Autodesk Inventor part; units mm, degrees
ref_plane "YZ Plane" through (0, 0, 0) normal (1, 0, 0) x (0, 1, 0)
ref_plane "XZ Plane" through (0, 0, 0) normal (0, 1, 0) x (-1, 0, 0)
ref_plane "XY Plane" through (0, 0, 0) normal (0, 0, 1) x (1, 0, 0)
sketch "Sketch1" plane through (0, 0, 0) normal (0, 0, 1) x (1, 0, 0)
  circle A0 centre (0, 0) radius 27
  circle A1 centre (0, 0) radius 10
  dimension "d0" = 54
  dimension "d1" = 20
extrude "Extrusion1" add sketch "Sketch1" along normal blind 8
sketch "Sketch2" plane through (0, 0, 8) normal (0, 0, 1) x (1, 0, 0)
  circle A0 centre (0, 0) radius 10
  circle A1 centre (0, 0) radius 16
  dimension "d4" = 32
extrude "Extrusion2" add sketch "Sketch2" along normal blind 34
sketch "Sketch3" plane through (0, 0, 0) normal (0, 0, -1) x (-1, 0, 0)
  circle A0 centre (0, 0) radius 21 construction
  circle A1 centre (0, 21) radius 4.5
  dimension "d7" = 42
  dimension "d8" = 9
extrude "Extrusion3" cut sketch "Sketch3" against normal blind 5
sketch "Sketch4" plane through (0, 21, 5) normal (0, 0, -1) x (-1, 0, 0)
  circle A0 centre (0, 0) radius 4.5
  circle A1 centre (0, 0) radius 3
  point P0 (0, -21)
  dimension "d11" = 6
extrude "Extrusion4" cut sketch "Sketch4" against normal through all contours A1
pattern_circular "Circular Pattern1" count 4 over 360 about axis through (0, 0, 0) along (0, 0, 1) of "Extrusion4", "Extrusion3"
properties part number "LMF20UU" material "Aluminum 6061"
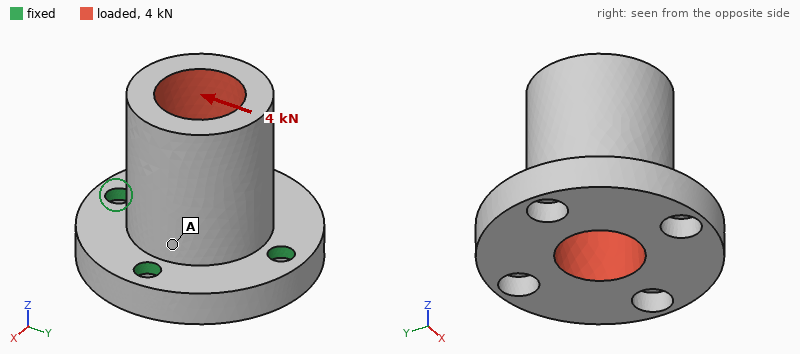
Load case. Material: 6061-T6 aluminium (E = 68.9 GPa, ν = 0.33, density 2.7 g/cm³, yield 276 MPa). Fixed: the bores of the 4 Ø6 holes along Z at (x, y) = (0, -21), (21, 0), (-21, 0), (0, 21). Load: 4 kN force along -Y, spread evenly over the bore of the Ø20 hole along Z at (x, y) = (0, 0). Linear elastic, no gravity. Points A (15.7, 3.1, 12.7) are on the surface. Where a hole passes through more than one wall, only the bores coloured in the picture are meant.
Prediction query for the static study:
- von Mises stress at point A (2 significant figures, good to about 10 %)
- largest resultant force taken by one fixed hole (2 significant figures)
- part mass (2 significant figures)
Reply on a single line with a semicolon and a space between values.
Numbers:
10 MPa; 1.7 kN; 83 g
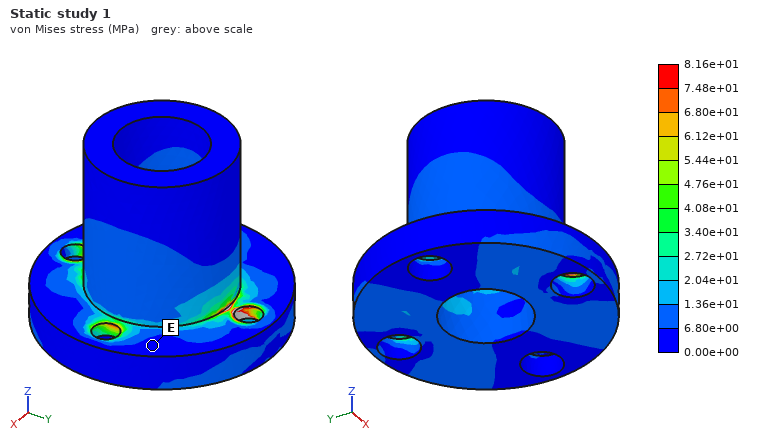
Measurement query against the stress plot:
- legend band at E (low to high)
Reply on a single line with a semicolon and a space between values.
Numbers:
0.00e+00 to 6.80e+00 MPa
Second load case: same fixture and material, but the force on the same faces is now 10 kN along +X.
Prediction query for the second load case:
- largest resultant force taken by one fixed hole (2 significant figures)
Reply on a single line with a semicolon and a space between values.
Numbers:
4.3 kN
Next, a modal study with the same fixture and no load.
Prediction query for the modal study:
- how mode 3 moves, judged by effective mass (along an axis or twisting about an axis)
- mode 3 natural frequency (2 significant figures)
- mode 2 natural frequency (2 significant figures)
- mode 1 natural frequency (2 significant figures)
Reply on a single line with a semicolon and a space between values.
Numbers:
along Z; 16 kHz; 8900 Hz; 8900 Hz
